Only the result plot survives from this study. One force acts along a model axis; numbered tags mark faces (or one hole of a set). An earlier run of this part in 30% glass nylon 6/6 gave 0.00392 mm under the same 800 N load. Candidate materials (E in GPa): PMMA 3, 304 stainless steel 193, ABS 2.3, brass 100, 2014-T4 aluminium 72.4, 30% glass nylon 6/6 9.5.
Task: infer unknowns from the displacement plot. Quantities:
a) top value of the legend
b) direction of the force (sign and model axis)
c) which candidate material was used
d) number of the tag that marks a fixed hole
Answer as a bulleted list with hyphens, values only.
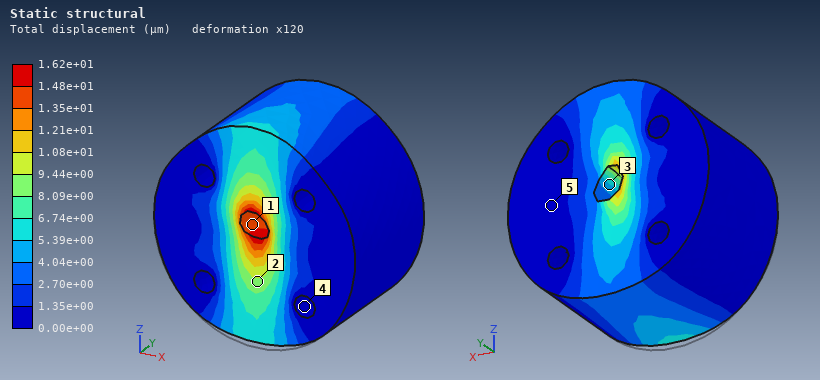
- 1.62e+01 µm
- +Z
- ABS
- 4
